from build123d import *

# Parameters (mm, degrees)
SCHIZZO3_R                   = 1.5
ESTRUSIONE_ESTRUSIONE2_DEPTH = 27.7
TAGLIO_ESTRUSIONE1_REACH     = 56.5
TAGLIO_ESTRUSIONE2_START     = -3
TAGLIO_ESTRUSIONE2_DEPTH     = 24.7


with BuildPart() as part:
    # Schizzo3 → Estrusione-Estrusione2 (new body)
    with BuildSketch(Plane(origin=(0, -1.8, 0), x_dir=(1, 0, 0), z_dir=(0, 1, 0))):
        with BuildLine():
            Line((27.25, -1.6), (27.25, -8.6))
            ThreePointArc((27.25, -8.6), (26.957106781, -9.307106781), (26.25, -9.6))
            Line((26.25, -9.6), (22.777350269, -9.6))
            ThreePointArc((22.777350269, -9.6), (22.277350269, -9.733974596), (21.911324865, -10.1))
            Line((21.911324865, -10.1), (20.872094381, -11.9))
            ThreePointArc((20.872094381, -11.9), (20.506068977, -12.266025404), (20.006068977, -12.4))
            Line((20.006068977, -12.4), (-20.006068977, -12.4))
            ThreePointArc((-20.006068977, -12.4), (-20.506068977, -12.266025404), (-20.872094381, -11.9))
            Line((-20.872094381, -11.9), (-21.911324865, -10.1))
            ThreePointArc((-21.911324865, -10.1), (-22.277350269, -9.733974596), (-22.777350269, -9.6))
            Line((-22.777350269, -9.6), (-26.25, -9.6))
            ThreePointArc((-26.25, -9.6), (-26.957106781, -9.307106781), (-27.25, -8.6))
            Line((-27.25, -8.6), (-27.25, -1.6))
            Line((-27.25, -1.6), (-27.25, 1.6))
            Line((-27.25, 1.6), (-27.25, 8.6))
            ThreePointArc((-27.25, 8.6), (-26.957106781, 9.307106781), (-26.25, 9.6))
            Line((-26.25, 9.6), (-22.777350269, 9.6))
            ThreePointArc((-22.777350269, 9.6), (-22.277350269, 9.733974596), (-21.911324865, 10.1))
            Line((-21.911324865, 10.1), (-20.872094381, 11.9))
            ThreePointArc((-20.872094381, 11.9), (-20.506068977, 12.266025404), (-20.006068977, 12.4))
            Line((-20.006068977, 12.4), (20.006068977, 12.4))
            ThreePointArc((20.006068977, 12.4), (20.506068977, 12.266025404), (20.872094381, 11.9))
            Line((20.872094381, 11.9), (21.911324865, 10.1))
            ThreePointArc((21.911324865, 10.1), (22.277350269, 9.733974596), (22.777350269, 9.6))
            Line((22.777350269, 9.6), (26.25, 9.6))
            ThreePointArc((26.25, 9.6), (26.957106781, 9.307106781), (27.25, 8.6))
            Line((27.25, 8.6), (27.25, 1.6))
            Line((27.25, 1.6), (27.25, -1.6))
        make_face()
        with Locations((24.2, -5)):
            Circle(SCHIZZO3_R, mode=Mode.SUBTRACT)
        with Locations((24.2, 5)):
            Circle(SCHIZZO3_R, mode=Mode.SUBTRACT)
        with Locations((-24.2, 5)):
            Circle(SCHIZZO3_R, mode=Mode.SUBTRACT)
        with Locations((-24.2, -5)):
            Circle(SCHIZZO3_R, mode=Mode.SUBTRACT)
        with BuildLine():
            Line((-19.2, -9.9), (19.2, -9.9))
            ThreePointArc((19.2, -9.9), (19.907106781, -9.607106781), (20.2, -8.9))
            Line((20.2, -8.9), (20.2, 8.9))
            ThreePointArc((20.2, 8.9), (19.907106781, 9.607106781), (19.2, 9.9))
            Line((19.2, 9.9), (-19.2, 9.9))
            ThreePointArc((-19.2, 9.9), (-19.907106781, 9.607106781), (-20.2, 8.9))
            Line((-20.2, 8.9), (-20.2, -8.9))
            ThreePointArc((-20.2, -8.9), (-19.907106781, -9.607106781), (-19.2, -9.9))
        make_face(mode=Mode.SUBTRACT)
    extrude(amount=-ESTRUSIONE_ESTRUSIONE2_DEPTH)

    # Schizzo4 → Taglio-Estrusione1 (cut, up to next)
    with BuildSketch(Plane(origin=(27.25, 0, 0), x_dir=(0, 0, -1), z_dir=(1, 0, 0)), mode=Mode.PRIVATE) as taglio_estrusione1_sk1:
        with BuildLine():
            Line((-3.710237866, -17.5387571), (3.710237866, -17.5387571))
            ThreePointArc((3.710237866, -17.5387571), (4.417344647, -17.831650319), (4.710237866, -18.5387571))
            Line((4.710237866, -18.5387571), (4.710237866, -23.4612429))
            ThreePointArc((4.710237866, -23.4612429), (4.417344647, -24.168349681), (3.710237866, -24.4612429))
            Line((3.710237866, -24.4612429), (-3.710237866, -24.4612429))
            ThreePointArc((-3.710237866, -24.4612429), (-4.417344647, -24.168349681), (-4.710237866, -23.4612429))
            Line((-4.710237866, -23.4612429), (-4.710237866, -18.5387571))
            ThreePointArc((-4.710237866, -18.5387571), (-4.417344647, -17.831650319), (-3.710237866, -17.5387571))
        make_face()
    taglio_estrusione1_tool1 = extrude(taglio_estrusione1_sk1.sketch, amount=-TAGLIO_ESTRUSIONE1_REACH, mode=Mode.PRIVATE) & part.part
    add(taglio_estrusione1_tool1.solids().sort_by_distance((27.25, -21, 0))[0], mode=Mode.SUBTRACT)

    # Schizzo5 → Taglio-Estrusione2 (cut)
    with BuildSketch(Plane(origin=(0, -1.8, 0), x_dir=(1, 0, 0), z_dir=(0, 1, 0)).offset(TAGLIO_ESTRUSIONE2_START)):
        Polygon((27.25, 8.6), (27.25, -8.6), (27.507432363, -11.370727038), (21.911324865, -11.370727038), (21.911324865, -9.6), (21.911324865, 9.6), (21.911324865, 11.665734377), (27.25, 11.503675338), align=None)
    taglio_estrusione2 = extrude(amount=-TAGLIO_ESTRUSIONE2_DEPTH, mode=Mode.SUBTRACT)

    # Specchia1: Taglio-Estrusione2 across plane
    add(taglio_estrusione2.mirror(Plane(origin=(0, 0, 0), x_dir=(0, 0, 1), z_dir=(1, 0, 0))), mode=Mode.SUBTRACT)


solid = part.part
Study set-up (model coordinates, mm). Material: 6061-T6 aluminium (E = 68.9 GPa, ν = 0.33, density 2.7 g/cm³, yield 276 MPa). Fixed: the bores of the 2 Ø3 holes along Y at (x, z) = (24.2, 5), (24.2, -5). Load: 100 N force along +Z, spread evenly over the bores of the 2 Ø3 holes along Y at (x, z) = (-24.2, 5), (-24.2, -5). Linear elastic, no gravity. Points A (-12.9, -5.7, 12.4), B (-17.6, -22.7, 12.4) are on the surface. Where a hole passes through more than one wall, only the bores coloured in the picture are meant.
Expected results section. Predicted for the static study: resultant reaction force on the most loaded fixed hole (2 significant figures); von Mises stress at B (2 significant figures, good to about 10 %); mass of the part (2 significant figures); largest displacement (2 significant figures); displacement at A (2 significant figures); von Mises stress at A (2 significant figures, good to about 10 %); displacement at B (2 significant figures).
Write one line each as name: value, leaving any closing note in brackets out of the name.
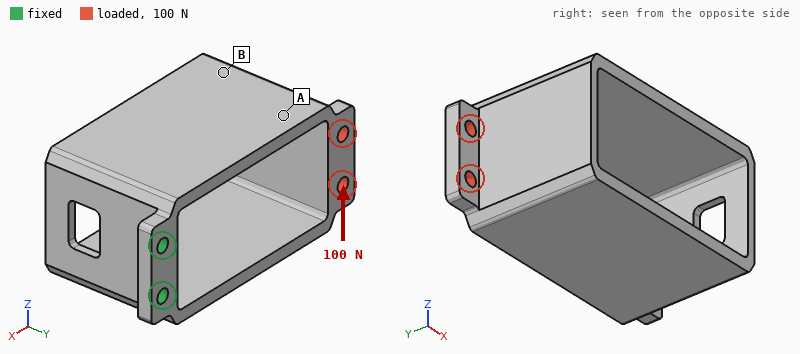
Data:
resultant reaction force on the most loaded fixed hole: 290 N
von Mises stress at B: 18 MPa
mass of the part: 22 g
largest displacement: 0.51 mm
displacement at A: 0.41 mm
von Mises stress at A: 34 MPa
displacement at B: 0.35 mm
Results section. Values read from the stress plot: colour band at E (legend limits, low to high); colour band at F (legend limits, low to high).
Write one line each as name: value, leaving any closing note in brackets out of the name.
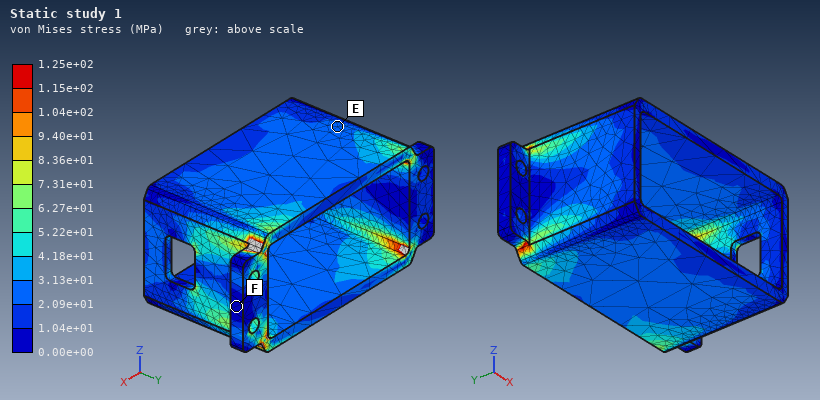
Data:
colour band at E: 2.09e+01 to 3.13e+01 MPa
colour band at F: 0.00e+00 to 1.04e+01 MPa
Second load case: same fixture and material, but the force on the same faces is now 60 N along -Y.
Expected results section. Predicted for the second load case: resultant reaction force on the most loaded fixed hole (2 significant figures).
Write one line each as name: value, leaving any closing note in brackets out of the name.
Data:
resultant reaction force on the most loaded fixed hole: 78 N
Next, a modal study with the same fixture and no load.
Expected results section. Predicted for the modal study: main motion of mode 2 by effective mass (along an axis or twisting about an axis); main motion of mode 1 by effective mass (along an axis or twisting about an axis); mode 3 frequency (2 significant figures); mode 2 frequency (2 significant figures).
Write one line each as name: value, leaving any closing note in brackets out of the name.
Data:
main motion of mode 2 by effective mass: along Z
main motion of mode 1 by effective mass: along Y
mode 3 frequency: 2200 Hz
mode 2 frequency: 860 Hz
